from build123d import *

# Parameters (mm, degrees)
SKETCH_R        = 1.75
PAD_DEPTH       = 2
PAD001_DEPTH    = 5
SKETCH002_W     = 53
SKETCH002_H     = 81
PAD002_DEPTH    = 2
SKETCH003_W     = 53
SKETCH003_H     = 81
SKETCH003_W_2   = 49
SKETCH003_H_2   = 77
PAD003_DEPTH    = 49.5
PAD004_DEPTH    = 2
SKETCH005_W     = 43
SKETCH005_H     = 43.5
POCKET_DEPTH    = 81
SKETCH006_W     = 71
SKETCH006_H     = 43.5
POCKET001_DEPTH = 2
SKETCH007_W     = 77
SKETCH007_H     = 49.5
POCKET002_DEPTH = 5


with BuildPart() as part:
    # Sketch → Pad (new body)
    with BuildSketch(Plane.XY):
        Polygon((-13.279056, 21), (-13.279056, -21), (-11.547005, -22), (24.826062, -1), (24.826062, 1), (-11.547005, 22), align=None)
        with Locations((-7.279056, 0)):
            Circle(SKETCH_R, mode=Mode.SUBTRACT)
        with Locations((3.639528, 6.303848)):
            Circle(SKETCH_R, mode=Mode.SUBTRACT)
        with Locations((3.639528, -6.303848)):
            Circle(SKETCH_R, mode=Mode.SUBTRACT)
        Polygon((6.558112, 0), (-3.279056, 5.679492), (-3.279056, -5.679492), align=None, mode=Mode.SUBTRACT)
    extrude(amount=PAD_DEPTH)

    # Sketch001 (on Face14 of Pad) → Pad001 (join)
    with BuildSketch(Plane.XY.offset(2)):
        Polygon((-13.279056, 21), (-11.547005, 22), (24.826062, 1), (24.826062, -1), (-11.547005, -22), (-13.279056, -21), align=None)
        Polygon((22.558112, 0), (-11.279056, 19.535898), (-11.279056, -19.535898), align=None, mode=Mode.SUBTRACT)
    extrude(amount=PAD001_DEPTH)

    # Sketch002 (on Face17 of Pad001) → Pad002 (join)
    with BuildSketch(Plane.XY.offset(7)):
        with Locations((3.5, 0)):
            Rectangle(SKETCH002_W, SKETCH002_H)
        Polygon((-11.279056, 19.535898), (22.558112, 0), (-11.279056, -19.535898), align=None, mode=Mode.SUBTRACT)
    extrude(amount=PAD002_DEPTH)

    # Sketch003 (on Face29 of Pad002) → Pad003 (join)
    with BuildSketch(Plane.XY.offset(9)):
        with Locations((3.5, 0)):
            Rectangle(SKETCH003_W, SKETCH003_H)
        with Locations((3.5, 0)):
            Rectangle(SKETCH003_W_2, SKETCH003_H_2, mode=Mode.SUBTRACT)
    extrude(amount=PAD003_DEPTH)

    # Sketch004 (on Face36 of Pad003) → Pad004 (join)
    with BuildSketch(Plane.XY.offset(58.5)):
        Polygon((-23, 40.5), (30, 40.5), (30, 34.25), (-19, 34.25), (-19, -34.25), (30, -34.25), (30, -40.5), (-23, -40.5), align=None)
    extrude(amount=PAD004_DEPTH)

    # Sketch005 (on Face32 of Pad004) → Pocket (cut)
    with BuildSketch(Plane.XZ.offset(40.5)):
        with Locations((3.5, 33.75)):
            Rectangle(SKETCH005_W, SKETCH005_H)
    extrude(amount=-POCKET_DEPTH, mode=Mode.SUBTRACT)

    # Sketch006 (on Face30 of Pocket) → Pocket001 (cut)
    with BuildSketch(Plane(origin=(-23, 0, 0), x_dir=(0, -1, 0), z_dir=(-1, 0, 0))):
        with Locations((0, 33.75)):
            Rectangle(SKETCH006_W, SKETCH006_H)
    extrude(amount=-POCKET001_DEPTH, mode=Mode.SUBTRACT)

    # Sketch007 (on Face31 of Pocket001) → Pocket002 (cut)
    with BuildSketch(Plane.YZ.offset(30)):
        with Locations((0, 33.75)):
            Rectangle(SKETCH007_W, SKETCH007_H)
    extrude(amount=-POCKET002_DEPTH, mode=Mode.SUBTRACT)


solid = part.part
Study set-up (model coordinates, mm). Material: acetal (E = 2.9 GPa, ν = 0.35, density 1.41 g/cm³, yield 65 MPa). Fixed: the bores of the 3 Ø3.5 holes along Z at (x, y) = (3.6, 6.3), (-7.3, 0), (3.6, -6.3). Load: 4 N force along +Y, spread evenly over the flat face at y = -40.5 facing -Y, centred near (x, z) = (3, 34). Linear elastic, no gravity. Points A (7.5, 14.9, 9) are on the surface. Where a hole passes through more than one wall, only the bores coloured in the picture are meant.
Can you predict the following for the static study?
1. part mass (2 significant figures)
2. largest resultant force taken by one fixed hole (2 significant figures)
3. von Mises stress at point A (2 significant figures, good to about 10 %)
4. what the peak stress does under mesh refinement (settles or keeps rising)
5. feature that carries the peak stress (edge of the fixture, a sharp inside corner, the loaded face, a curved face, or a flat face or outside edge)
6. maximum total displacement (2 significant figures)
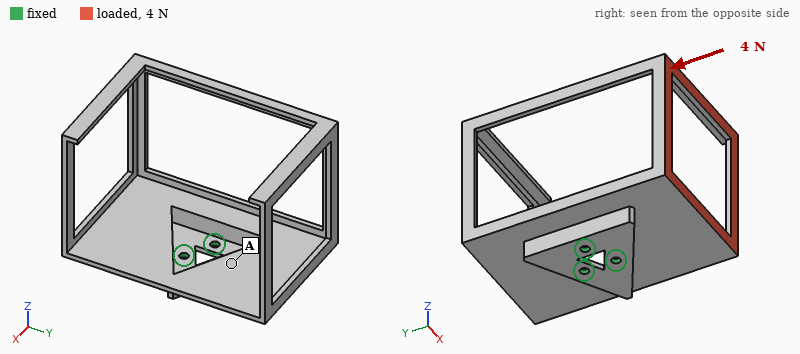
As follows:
23 g
5.9 N
0.43 MPa
keeps rising
a sharp inside corner
1.1 mm
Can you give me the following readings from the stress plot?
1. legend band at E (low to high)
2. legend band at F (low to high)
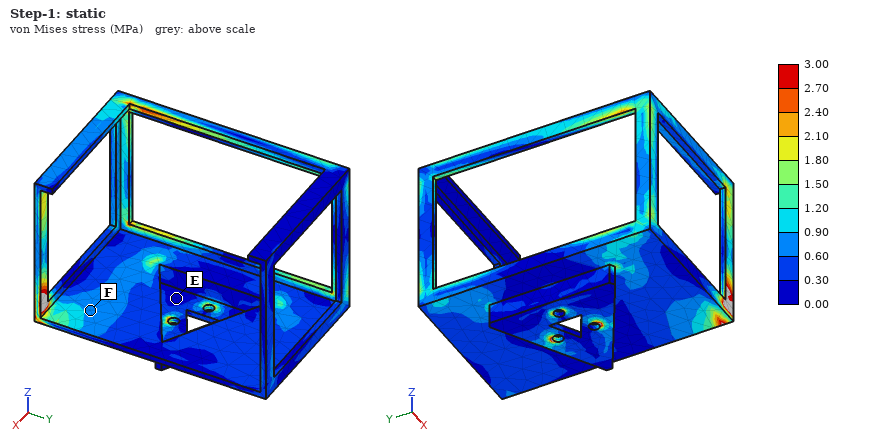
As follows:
0.00 to 0.30 MPa
0.60 to 0.90 MPa
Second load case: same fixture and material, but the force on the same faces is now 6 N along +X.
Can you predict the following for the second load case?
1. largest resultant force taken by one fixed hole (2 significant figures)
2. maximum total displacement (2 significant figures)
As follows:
17 N
1.1 mm
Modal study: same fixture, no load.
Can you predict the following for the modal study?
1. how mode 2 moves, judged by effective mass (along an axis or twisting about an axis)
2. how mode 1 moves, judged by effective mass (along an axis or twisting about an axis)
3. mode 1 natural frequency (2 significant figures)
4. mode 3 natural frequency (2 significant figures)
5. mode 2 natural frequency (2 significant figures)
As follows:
along X
along Y
130 Hz
210 Hz
140 Hz
